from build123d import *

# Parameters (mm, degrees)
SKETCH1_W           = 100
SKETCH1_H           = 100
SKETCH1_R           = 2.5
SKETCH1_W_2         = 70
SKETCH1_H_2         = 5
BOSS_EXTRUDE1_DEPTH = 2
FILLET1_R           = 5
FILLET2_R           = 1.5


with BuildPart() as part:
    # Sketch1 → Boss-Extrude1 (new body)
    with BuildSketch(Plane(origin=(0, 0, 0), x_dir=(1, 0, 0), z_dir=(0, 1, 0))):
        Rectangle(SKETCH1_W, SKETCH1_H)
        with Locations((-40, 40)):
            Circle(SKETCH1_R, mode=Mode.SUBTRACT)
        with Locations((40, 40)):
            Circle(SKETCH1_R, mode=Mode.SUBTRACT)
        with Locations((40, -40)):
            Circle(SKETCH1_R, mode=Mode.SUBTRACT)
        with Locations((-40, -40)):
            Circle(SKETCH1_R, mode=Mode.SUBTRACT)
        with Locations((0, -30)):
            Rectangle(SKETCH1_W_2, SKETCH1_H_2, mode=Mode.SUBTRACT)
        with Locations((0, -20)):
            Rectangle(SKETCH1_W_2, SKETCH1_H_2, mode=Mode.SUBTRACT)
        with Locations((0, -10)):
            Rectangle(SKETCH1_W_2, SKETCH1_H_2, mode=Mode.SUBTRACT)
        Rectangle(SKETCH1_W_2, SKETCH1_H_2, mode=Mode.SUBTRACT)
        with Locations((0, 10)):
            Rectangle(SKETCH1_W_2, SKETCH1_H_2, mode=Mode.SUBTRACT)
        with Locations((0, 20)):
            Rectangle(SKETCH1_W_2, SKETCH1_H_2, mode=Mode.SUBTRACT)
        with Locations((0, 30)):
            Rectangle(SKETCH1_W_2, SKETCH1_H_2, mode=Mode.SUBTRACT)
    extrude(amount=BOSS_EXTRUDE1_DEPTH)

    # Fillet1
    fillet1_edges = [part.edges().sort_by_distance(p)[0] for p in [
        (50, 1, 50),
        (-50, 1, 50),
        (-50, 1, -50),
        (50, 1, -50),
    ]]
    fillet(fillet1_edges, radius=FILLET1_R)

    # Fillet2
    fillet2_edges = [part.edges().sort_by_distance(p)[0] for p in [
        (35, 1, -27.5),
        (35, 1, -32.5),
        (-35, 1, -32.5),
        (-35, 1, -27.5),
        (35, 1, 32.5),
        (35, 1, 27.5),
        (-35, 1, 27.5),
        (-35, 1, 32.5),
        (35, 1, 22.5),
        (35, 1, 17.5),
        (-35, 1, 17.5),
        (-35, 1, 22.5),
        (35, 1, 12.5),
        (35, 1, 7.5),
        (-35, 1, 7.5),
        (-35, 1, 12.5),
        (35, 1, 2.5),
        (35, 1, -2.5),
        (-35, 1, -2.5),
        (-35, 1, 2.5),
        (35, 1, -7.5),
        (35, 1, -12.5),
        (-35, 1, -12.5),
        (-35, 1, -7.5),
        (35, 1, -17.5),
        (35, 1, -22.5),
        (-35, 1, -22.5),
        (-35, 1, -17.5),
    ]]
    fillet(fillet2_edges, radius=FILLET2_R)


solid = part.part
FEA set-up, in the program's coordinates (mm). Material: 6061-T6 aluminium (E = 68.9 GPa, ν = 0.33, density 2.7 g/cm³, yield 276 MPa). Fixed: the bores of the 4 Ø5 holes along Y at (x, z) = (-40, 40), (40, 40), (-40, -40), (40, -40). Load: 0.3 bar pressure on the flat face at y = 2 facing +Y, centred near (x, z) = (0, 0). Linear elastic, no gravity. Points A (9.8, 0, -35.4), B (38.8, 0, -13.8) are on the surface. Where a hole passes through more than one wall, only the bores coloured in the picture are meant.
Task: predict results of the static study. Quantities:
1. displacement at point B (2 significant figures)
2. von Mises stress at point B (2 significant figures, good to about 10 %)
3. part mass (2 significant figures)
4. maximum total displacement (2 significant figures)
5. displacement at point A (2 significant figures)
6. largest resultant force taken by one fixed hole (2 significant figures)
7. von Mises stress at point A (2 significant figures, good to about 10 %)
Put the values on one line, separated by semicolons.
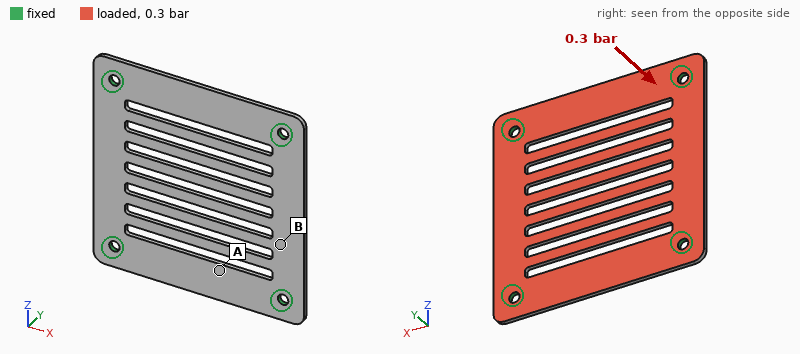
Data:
0.096 mm; 18 MPa; 40 g; 0.27 mm; 0.052 mm; 56 N; 8.1 MPa
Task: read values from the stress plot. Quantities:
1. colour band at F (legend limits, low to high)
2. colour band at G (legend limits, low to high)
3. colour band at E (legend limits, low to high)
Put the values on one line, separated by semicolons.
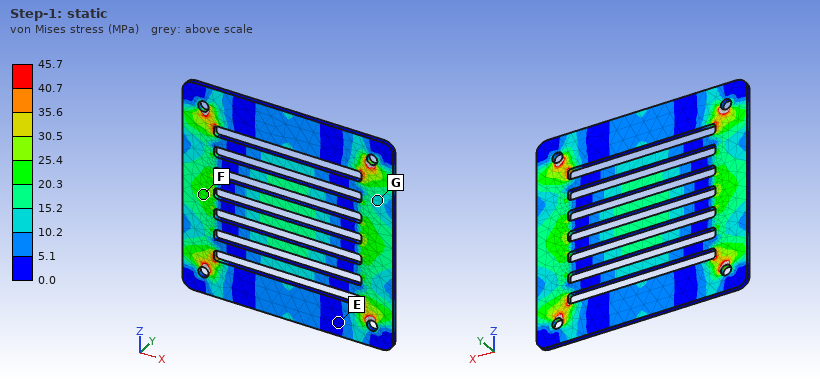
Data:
20.3 to 25.4 MPa; 10.2 to 15.2 MPa; 0.0 to 5.1 MPa
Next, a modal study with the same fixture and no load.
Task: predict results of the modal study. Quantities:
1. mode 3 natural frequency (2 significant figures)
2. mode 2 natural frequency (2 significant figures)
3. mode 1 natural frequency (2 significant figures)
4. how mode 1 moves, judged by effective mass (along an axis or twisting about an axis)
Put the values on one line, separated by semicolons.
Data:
1600 Hz; 1400 Hz; 910 Hz; along Y
